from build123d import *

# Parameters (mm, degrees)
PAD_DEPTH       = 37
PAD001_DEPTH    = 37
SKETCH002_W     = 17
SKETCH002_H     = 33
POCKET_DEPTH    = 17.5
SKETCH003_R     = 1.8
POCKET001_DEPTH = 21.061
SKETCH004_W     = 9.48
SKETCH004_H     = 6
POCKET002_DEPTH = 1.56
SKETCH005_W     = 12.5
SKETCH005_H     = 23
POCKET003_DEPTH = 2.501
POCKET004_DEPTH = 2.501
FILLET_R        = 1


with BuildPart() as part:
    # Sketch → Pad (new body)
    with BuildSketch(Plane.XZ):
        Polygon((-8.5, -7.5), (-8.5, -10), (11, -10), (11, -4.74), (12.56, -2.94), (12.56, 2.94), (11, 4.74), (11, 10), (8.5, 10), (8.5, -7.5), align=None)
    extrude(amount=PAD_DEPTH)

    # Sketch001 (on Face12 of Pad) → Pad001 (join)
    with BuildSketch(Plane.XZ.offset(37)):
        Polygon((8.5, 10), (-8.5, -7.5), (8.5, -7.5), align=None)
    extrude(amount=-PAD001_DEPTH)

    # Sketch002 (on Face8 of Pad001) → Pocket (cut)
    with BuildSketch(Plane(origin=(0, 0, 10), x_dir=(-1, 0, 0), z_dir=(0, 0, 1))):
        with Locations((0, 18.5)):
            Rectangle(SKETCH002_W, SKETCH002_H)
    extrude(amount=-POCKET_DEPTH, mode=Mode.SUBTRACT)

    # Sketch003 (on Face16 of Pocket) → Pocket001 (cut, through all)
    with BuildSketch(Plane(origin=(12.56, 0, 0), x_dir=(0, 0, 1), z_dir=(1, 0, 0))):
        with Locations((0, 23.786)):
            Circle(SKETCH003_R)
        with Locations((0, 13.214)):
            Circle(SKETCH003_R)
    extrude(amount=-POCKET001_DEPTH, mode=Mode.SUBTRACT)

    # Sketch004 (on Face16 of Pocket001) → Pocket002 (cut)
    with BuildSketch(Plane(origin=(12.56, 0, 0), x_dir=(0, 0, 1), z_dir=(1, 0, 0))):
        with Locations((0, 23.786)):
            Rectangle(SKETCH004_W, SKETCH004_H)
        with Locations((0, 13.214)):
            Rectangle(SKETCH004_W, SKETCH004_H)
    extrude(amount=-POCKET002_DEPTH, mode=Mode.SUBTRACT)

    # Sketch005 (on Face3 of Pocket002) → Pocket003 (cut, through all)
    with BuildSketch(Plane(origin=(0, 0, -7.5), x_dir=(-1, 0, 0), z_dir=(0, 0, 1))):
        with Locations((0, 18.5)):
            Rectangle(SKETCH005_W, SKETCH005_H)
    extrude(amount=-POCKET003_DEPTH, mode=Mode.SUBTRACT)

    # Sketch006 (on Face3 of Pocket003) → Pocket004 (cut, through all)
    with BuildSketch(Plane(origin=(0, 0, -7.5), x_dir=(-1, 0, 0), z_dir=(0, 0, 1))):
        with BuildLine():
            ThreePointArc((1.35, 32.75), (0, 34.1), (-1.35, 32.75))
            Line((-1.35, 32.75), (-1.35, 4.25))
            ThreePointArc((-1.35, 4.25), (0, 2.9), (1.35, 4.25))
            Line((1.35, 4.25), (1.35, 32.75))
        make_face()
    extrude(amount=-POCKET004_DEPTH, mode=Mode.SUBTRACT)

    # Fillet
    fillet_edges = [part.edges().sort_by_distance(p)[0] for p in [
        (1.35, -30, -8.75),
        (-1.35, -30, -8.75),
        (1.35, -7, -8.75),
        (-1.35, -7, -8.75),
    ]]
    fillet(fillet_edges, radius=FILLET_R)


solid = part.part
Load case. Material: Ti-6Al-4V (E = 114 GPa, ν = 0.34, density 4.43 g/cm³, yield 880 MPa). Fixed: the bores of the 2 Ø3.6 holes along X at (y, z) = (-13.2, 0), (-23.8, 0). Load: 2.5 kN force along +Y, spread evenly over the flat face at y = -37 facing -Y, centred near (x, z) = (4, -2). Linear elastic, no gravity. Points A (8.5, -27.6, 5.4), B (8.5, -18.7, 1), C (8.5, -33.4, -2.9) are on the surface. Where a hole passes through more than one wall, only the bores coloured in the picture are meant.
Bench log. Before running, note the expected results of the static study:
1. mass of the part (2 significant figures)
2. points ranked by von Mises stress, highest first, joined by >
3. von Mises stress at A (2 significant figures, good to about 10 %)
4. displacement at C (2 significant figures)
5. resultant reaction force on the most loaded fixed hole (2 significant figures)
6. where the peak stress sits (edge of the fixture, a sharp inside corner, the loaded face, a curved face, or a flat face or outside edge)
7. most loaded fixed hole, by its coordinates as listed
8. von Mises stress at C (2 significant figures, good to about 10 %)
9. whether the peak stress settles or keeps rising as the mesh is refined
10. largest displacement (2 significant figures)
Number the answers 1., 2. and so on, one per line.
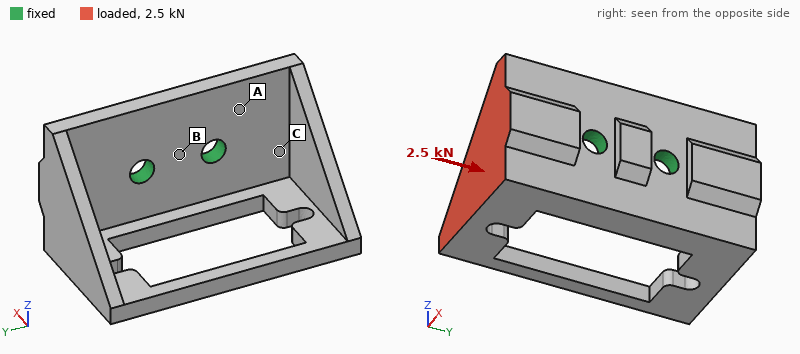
1. 15 g
2. A > C > B
3. 230 MPa
4. 0.082 mm
5. 1.8 kN
6. edge of the fixture
7. (-23.8, 0)
8. 150 MPa
9. keeps rising
10. 0.29 mm
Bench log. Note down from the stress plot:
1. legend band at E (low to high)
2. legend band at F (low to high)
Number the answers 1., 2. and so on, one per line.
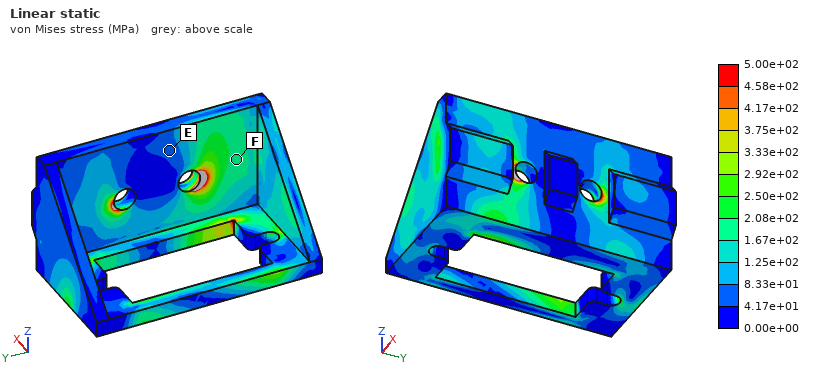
1. 4.17e+01 to 8.33e+01 MPa
2. 1.67e+02 to 2.08e+02 MPa
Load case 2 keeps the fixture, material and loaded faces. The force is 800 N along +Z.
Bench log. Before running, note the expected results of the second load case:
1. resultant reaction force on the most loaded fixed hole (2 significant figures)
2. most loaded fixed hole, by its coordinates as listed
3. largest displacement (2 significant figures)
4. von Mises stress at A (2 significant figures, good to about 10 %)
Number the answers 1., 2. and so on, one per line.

1. 1.5 kN
2. (-23.8, 0)
3. 0.15 mm
4. 87 MPa
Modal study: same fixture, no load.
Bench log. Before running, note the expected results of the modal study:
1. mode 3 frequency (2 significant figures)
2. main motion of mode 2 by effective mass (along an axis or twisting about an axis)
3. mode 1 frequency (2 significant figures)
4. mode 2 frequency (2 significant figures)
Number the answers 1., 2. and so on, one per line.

1. 7800 Hz
2. along Z
3. 4900 Hz
4. 5500 Hz
